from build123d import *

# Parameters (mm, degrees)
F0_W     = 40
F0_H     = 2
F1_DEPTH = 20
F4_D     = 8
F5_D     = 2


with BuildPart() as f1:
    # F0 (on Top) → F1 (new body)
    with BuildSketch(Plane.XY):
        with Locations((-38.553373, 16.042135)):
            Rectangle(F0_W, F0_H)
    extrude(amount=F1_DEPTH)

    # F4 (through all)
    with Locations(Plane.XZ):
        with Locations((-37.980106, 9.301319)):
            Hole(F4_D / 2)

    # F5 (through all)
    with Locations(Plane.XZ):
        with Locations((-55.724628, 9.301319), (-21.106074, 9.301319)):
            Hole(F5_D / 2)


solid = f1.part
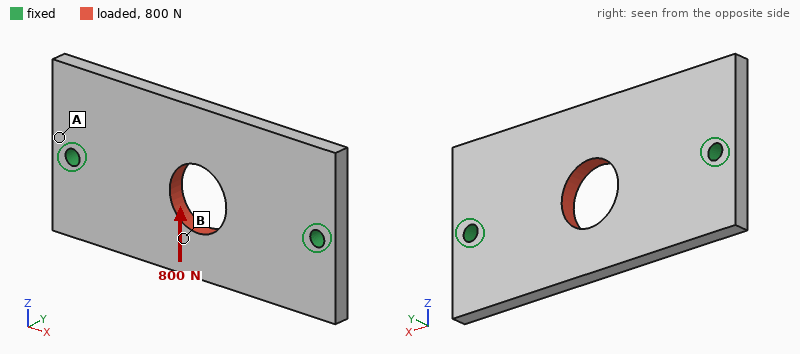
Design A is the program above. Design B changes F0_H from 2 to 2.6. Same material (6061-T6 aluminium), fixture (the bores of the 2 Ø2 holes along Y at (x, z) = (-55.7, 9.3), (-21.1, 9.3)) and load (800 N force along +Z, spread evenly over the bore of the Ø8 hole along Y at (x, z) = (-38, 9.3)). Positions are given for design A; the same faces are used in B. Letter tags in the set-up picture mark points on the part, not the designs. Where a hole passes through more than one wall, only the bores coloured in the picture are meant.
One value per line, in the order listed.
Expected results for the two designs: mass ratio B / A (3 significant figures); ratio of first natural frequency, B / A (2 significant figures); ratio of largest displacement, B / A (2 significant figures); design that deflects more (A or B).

1.30
1.2
0.77
A
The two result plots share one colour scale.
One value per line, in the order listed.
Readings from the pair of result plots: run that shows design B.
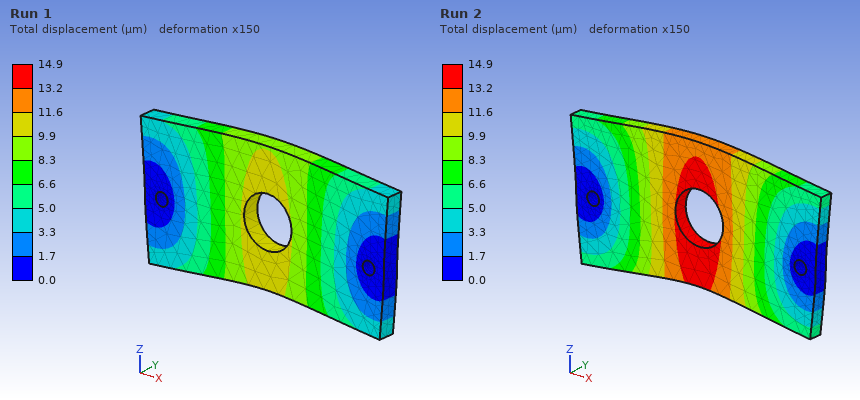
Run 1
